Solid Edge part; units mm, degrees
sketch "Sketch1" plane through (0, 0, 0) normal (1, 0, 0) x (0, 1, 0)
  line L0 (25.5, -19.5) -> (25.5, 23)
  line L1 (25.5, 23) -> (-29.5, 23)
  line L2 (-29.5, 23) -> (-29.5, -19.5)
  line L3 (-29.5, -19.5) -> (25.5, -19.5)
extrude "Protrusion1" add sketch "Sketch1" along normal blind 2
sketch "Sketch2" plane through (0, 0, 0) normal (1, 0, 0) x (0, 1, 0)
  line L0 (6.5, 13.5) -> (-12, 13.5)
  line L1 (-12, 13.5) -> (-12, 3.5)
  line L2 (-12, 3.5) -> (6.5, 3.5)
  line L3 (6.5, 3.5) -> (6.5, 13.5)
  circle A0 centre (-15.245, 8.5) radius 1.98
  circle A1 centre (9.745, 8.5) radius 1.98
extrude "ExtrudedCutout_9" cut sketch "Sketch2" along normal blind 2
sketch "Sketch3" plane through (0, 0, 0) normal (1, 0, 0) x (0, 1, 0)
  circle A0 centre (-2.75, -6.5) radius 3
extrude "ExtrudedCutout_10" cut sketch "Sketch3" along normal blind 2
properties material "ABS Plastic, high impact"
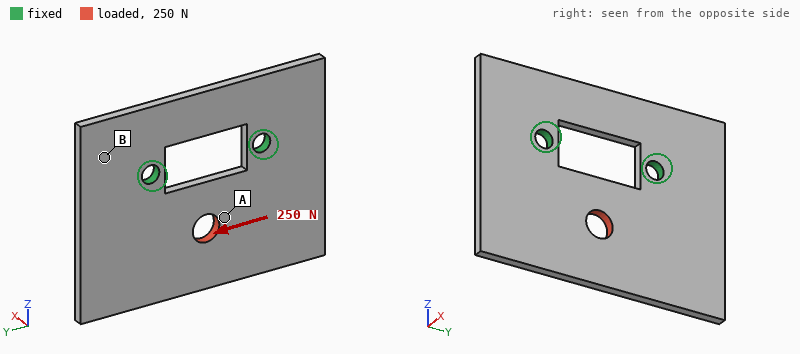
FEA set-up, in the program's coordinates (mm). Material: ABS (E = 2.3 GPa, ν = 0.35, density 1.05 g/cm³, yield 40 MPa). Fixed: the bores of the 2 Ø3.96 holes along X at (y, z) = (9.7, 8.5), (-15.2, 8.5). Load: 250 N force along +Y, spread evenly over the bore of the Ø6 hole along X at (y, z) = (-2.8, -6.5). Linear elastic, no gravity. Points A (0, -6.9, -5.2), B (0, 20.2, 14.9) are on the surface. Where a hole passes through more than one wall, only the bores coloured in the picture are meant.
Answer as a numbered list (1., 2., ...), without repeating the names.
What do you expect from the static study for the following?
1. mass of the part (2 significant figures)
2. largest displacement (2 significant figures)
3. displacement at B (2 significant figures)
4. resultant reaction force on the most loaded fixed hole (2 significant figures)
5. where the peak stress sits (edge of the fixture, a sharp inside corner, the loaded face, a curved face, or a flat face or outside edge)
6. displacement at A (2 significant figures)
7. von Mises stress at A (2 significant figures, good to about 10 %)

1. 4.4 g
2. 0.20 mm
3. 0.065 mm
4. 170 N
5. edge of the fixture
6. 0.12 mm
7. 8.9 MPa
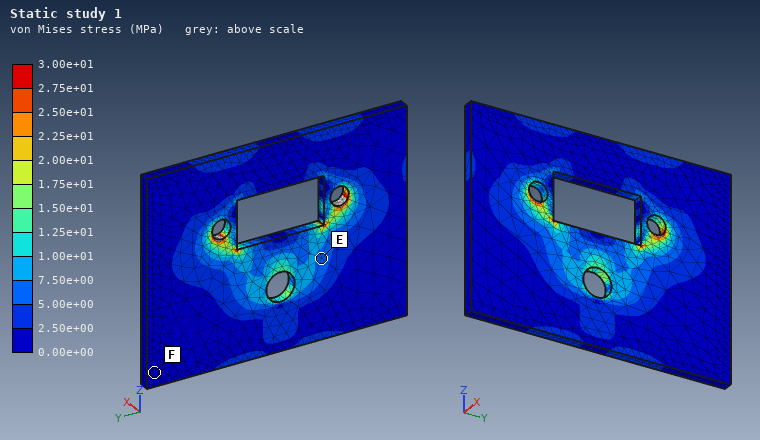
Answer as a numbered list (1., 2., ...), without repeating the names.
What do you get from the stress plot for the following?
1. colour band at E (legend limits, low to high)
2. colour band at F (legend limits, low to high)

1. 5.00e+00 to 7.50e+00 MPa
2. 0.00e+00 to 2.50e+00 MPa
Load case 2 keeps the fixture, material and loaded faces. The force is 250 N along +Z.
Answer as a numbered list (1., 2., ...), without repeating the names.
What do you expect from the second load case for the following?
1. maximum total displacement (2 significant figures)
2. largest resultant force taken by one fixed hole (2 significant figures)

1. 84 µm
2. 130 N
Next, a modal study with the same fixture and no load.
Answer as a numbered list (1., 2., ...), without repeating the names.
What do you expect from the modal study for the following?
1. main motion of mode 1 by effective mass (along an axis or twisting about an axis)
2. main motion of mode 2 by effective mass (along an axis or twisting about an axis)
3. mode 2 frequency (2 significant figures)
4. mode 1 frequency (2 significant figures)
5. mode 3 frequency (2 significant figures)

1. along X
2. twisting about Z
3. 820 Hz
4. 520 Hz
5. 1400 Hz
